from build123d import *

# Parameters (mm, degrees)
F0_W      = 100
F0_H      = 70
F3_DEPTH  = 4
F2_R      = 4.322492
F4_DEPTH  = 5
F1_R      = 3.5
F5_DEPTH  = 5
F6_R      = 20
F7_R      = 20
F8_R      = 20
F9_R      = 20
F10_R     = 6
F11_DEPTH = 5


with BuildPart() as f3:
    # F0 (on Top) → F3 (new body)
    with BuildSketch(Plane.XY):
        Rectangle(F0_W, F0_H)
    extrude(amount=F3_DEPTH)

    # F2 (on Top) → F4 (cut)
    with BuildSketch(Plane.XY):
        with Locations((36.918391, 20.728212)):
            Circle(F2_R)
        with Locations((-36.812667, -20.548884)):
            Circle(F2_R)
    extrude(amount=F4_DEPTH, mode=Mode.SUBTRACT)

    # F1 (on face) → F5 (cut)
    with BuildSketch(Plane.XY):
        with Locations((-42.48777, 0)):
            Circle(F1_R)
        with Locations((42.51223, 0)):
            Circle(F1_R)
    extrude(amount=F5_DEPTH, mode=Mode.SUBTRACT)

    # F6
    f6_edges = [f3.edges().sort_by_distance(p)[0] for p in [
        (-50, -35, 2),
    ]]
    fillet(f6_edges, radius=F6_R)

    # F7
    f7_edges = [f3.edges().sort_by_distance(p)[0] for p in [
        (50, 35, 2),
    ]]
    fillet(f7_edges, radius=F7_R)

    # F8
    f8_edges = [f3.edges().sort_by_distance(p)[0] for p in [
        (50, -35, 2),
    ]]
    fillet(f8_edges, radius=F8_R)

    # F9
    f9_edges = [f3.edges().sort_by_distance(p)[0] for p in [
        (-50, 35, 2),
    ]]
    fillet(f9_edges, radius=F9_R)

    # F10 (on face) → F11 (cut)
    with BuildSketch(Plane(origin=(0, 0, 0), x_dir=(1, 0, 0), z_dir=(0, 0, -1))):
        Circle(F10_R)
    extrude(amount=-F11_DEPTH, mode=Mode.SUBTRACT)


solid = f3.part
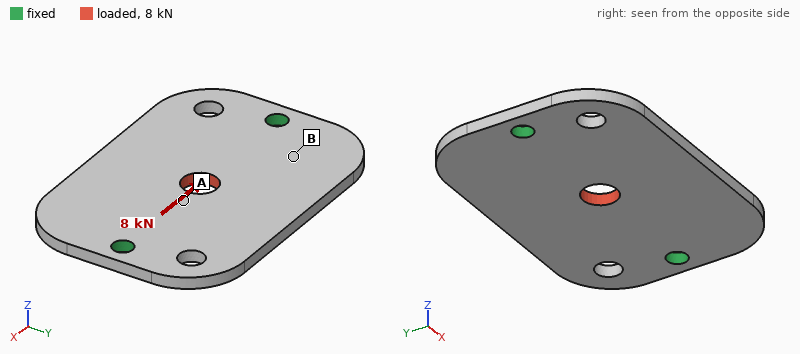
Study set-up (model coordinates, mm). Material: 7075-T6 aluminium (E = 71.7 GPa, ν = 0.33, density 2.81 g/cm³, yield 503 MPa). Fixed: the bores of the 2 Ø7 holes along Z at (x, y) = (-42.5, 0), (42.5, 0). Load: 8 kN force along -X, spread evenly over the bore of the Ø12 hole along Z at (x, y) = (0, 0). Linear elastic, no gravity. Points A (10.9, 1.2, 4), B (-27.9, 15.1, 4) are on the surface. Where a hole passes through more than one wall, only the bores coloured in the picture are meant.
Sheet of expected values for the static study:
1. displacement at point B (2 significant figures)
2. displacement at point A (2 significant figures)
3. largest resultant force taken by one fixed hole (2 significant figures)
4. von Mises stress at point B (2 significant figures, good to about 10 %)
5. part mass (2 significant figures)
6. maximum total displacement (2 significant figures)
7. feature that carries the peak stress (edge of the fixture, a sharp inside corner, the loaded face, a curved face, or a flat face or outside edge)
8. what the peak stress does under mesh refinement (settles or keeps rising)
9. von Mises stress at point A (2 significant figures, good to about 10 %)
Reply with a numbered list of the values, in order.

1. 12 µm
2. 19 µm
3. 4.0 kN
4. 16 MPa
5. 71 g
6. 24 µm
7. edge of the fixture
8. keeps rising
9. 51 MPa
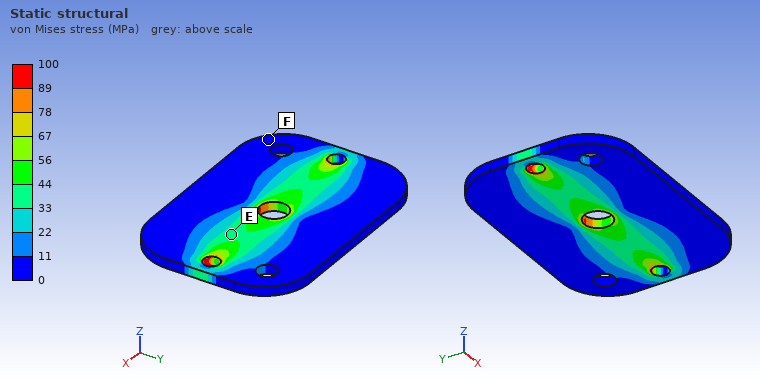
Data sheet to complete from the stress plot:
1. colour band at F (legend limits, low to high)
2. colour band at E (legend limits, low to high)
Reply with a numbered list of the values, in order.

1. 0 to 11 MPa
2. 33 to 44 MPa
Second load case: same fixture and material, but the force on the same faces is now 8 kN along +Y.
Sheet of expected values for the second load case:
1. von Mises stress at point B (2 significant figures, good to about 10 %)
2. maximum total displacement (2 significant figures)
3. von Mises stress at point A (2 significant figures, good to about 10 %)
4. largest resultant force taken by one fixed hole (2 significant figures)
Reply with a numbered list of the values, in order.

1. 32 MPa
2. 44 µm
3. 37 MPa
4. 4.0 kN
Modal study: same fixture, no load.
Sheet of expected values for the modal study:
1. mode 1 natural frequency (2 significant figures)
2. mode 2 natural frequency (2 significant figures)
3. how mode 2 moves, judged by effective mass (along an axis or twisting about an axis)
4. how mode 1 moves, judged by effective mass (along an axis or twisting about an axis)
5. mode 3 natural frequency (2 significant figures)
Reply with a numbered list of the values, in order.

1. 1700 Hz
2. 2000 Hz
3. along Z
4. twisting about X
5. 3800 Hz
